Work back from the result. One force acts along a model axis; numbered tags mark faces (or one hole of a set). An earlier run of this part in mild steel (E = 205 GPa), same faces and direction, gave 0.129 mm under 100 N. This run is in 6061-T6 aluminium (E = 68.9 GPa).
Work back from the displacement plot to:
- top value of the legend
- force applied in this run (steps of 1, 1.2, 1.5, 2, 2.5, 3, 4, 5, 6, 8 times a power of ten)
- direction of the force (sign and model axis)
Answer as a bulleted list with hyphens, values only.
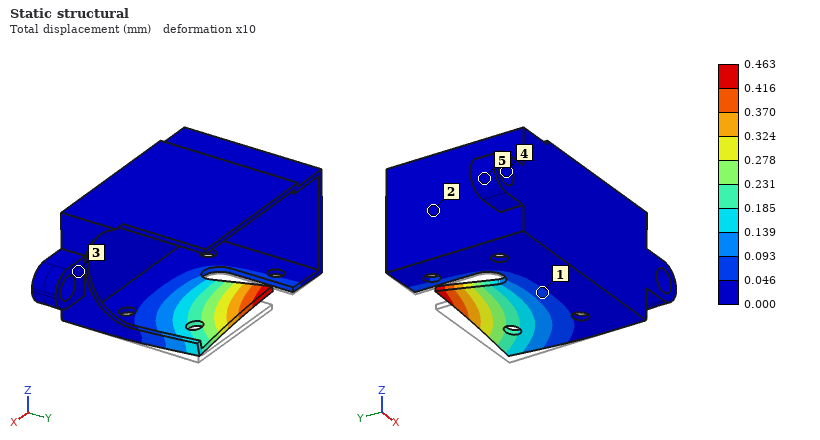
- 0.463 mm
- 120 N
- +Z
